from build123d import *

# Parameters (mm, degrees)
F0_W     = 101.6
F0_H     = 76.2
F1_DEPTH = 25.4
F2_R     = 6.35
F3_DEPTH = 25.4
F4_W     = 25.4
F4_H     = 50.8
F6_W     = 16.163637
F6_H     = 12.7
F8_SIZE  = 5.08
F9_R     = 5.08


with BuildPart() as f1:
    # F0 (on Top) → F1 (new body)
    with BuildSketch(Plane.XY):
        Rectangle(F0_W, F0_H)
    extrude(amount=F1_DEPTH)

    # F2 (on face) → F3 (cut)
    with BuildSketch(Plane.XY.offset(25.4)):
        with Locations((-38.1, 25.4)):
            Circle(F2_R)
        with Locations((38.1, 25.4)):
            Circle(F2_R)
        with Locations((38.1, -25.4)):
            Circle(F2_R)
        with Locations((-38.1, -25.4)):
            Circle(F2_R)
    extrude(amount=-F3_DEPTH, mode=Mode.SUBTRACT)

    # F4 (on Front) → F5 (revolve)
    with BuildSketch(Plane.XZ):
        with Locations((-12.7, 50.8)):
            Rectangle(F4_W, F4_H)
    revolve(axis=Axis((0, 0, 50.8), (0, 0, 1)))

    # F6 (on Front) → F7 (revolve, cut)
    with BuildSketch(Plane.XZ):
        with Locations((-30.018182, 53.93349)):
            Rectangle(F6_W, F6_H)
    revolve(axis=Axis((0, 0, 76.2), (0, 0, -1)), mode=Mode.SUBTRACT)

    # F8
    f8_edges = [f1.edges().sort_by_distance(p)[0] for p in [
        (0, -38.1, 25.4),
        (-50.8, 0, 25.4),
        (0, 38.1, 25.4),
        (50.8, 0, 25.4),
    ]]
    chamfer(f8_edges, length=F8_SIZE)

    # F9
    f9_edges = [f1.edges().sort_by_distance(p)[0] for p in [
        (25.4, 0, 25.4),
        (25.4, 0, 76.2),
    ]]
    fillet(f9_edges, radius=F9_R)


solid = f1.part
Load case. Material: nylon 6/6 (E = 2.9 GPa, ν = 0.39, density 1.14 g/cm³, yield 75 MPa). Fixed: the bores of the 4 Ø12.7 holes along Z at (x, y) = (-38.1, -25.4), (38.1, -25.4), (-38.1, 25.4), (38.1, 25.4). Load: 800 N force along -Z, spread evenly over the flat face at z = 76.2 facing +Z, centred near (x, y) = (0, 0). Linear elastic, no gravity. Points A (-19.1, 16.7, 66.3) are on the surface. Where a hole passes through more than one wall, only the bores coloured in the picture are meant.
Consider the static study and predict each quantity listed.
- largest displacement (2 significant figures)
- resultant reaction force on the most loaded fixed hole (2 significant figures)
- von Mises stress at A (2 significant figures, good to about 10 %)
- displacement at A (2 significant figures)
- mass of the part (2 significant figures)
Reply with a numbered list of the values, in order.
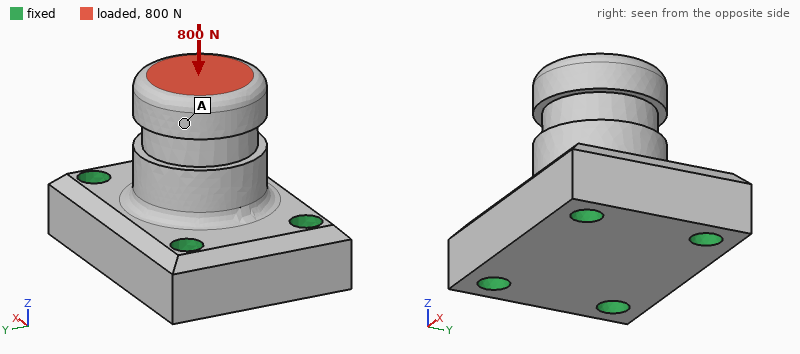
1. 16 µm
2. 210 N
3. 0.18 MPa
4. 13 µm
5. 310 g
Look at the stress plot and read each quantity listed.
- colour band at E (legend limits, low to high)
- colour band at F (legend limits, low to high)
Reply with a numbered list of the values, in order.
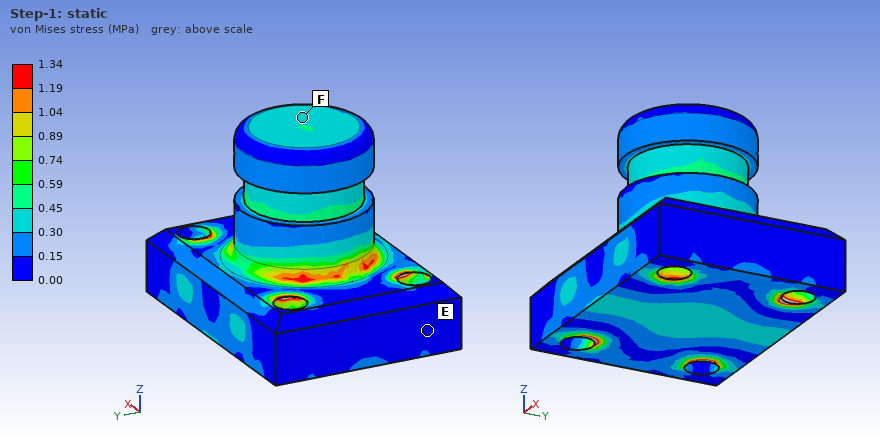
1. 0.00 to 0.15 MPa
2. 0.30 to 0.45 MPa
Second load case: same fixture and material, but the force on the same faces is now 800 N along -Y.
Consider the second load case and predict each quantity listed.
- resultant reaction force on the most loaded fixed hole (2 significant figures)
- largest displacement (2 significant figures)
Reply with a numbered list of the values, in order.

1. 530 N
2. 0.13 mm
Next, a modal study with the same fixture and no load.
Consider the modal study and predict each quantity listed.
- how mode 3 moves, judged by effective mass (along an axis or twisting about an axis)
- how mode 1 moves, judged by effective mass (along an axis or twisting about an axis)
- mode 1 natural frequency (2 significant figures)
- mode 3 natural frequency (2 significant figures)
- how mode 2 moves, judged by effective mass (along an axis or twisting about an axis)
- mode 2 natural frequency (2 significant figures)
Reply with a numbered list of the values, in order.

1. along Z
2. along Y
3. 2000 Hz
4. 3500 Hz
5. along X
6. 2400 Hz
